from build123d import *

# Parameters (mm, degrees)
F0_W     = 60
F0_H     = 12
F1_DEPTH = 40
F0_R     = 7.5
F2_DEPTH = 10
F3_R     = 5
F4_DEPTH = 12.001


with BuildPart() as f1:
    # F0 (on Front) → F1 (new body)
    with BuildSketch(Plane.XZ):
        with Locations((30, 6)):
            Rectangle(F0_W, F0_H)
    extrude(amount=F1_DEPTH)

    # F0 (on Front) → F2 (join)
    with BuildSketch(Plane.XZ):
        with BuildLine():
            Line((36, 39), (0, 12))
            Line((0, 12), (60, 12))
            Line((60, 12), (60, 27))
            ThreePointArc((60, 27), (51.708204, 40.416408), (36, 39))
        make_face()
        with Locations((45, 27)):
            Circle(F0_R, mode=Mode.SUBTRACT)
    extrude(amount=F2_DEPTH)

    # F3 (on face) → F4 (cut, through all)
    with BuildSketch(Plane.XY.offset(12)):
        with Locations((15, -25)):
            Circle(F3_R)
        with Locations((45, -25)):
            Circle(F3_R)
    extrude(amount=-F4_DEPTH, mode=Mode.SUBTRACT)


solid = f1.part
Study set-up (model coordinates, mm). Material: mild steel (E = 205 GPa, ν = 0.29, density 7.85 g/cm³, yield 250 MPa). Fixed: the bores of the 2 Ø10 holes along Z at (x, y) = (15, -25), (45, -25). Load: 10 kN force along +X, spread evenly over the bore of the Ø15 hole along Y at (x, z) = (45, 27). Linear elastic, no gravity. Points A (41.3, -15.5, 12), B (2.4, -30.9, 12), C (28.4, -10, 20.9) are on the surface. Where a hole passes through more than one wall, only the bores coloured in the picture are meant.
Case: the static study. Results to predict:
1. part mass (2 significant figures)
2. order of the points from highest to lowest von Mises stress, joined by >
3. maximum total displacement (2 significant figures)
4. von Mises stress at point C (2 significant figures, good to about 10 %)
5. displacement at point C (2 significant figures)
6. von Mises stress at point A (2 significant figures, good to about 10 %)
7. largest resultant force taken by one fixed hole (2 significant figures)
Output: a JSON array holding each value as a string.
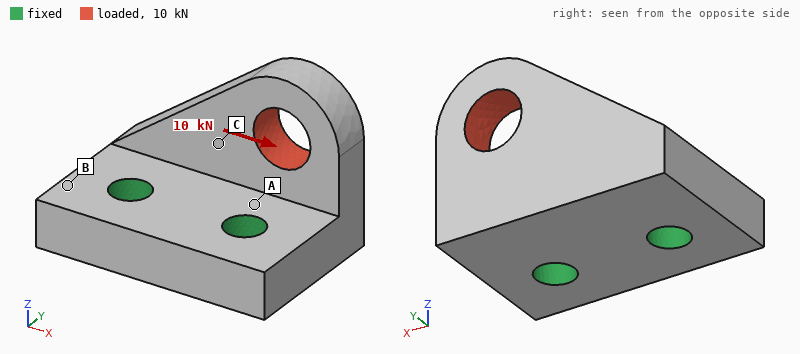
["290 g", "A > C > B", "42 µm", "45 MPa", "15 µm", "87 MPa", "8.5 kN"]
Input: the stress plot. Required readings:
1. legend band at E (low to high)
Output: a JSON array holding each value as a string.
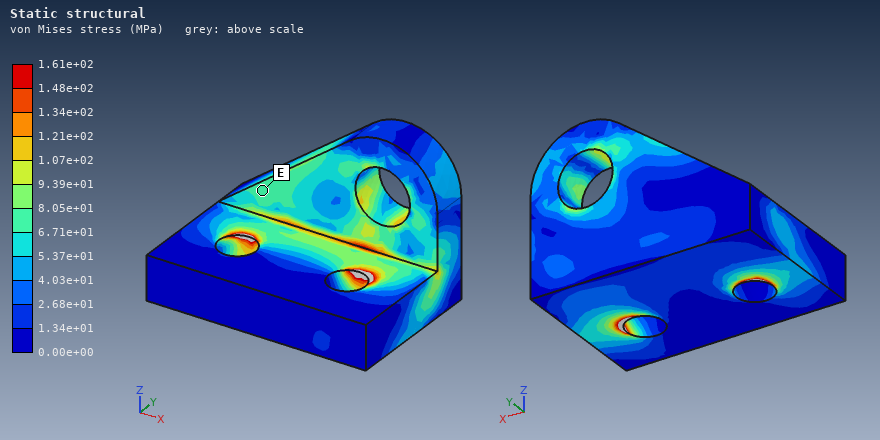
["6.71e+01 to 8.05e+01 MPa"]
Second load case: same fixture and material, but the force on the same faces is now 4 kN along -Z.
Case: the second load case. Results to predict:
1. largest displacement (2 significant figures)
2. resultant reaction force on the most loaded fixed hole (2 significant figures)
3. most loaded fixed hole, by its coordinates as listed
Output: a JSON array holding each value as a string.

["24 µm", "3.5 kN", "(45, -25)"]
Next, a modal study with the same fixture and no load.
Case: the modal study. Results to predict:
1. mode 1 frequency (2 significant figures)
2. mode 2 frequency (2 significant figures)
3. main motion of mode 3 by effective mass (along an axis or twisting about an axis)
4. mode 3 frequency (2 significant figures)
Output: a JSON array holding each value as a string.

["6200 Hz", "10 kHz", "along Z", "13 kHz"]
